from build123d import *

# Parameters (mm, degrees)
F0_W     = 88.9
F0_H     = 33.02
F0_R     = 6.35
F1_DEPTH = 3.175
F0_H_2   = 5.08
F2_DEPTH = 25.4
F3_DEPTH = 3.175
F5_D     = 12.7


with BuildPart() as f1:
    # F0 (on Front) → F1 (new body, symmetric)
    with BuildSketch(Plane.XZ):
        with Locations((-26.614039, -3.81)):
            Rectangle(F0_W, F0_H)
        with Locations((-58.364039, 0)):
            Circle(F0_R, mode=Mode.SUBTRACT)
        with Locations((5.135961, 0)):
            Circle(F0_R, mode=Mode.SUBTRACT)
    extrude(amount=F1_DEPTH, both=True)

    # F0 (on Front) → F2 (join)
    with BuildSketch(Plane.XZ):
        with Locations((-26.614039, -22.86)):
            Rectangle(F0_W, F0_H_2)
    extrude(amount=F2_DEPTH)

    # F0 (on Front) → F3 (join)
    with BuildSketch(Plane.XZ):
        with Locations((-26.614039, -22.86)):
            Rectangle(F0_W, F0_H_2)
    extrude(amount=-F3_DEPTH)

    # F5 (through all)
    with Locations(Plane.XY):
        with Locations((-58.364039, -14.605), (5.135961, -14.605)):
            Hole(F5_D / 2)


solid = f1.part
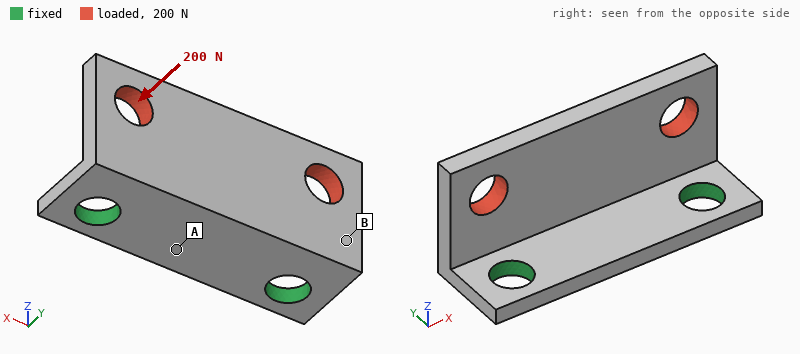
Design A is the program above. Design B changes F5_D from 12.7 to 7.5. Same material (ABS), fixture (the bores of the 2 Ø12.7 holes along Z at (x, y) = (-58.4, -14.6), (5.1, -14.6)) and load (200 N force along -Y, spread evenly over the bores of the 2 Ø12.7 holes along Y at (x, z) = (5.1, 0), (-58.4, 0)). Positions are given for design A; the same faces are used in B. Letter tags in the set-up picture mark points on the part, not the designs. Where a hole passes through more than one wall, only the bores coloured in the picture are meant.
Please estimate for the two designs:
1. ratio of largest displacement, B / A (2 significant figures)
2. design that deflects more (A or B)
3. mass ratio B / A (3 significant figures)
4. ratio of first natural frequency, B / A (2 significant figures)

1.3
B
1.03
0.86
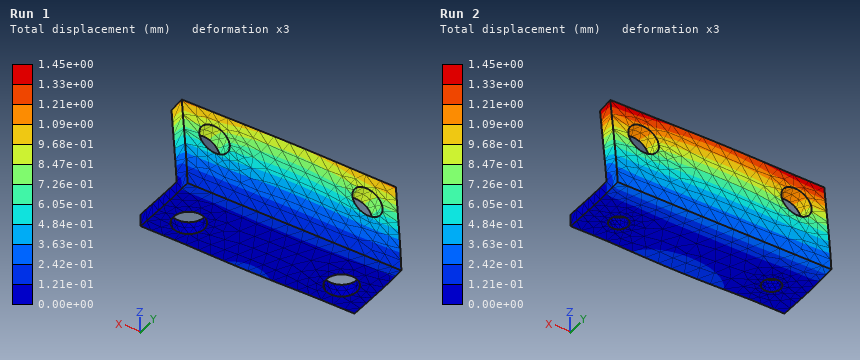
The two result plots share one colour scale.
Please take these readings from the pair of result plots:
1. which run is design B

Run 2
